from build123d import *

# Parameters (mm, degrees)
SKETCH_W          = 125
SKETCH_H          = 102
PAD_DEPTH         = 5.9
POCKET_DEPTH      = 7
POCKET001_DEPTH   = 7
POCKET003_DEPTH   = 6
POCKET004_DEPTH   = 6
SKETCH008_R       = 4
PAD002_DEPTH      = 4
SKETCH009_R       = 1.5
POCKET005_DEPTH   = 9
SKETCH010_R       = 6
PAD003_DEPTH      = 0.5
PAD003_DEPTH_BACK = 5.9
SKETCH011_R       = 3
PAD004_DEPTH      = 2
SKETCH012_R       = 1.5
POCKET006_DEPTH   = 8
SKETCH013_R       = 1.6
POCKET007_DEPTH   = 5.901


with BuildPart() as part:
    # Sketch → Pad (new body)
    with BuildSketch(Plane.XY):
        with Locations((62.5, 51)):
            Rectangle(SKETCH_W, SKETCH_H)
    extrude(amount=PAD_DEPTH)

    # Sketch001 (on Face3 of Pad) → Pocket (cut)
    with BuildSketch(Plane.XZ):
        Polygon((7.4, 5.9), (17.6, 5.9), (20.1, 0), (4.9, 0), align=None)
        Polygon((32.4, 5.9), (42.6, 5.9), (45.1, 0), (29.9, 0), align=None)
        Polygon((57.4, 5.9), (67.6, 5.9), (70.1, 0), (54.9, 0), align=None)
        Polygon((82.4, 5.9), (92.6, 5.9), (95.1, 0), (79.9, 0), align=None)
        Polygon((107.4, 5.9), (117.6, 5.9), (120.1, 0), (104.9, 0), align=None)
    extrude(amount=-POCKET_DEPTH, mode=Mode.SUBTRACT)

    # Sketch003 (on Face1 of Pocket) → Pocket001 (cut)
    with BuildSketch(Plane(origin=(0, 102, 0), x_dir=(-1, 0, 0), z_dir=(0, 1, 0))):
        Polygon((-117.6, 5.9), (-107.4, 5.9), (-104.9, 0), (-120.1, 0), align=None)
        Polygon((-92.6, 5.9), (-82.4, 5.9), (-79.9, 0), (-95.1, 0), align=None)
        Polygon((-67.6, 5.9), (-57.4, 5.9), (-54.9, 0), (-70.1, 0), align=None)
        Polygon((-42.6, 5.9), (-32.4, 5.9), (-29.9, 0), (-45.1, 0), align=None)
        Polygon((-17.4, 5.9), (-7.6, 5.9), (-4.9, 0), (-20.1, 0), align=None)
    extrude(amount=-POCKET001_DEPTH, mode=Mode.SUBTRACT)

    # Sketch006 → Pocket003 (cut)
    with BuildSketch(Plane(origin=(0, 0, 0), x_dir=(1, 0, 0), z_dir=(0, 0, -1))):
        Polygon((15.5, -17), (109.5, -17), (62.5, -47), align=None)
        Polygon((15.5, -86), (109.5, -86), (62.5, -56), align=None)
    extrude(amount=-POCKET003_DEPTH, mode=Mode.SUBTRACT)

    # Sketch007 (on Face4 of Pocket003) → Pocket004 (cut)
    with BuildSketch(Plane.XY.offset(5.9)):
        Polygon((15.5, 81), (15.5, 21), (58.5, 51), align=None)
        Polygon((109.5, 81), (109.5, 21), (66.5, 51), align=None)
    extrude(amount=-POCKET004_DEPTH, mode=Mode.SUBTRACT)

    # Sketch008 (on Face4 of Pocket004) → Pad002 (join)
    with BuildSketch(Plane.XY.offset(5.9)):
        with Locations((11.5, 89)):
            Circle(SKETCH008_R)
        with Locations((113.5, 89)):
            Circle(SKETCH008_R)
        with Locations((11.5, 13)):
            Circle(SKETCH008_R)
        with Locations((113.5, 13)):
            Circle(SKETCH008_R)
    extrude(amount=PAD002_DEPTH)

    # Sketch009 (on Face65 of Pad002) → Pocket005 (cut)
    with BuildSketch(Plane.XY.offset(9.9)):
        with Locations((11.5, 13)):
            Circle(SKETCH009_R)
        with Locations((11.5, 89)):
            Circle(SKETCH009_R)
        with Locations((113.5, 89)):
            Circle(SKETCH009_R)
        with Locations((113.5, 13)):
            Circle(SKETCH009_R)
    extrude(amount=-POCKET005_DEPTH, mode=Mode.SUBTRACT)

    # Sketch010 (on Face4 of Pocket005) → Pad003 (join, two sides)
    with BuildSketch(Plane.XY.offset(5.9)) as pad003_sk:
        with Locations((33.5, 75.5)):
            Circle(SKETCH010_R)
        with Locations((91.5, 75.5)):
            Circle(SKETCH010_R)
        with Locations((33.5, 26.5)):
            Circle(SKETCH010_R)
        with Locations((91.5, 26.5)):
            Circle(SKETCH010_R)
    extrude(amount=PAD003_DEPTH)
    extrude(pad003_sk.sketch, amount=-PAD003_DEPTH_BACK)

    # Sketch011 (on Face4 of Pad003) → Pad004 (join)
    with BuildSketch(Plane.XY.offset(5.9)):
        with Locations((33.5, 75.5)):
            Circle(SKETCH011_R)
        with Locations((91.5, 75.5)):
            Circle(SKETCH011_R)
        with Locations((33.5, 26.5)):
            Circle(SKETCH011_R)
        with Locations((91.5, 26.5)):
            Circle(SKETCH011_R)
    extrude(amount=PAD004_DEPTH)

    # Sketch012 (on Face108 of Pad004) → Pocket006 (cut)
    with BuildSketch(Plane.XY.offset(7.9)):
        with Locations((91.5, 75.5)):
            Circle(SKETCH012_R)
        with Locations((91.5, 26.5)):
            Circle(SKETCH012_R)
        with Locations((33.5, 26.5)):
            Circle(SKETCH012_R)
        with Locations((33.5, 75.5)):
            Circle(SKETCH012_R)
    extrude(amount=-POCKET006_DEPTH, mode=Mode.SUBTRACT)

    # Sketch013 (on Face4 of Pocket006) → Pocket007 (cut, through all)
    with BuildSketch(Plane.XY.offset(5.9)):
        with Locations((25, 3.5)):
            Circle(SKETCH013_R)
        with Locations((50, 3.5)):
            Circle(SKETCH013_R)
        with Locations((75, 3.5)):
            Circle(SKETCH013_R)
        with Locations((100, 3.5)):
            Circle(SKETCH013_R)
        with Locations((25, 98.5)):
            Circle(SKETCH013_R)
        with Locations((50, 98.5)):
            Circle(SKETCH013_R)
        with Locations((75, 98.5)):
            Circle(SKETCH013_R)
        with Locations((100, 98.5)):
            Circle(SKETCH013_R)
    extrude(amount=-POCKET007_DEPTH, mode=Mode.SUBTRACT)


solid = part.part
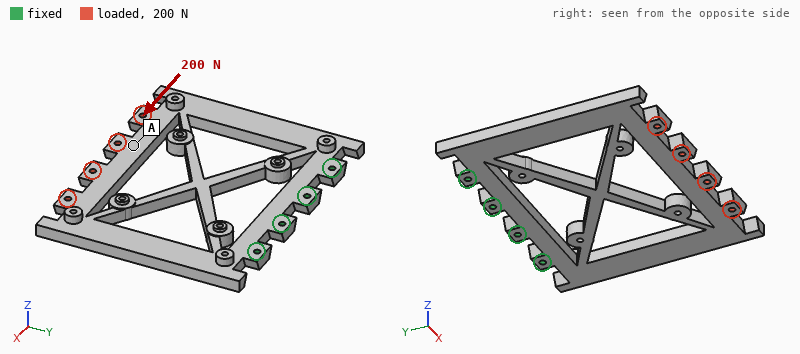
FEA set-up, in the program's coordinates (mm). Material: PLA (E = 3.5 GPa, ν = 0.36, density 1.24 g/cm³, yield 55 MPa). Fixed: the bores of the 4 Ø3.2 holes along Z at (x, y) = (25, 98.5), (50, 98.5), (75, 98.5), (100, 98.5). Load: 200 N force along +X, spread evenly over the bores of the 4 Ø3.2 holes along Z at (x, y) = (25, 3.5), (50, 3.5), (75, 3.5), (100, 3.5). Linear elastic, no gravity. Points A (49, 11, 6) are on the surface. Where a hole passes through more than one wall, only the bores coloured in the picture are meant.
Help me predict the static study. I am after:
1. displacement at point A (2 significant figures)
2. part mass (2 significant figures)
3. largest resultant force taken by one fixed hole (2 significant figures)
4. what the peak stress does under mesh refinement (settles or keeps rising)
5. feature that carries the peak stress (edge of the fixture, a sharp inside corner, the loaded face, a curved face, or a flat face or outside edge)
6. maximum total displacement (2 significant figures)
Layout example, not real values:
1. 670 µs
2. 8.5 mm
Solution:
1. 0.53 mm
2. 50 g
3. 250 N
4. keeps rising
5. edge of the fixture
6. 0.60 mm
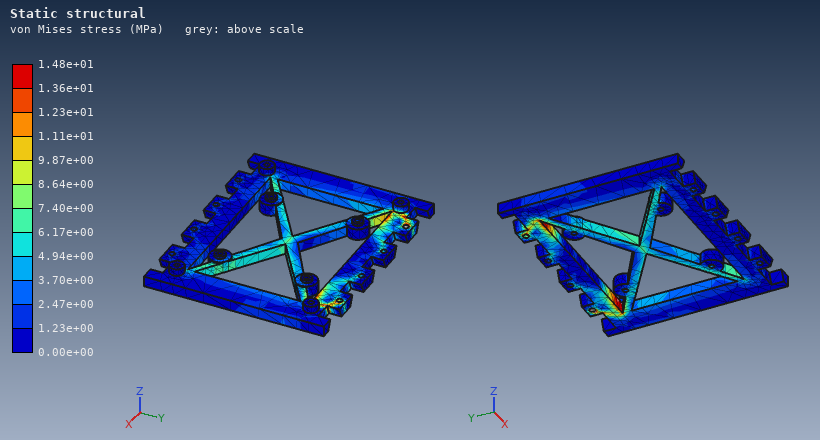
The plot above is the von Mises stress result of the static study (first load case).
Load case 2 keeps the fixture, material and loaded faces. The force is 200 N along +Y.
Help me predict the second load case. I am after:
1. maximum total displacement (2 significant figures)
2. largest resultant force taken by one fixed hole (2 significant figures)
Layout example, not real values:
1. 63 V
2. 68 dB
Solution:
1. 0.64 mm
2. 140 N
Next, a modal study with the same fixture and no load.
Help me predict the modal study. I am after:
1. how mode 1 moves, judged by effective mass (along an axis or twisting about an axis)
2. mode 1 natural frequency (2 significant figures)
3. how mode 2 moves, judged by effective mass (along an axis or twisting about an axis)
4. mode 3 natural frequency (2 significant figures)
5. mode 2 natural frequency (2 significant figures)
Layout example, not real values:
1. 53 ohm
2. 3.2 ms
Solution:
1. along Z
2. 89 Hz
3. twisting about Y
4. 530 Hz
5. 200 Hz
